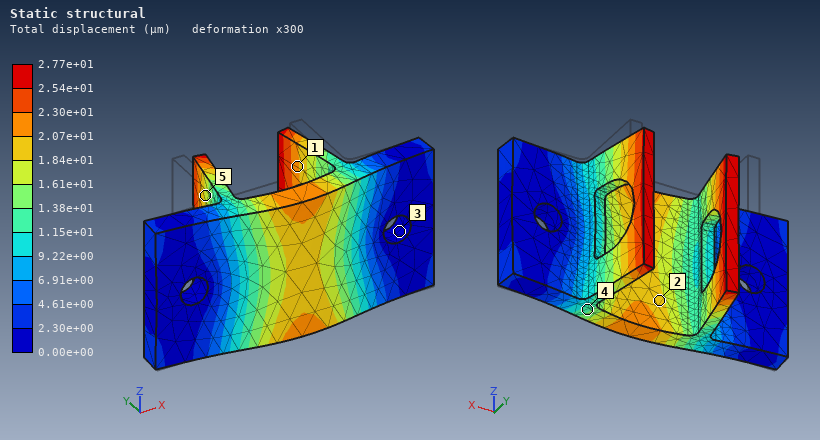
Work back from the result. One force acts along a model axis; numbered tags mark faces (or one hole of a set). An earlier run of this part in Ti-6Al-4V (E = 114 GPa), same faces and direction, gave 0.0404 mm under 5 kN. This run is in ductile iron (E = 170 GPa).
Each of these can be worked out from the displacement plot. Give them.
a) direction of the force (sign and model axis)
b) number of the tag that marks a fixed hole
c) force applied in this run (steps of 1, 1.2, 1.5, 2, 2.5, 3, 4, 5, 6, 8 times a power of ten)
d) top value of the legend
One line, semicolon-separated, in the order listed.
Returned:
-Y; 3; 5 kN; 2.77e+01 µm
